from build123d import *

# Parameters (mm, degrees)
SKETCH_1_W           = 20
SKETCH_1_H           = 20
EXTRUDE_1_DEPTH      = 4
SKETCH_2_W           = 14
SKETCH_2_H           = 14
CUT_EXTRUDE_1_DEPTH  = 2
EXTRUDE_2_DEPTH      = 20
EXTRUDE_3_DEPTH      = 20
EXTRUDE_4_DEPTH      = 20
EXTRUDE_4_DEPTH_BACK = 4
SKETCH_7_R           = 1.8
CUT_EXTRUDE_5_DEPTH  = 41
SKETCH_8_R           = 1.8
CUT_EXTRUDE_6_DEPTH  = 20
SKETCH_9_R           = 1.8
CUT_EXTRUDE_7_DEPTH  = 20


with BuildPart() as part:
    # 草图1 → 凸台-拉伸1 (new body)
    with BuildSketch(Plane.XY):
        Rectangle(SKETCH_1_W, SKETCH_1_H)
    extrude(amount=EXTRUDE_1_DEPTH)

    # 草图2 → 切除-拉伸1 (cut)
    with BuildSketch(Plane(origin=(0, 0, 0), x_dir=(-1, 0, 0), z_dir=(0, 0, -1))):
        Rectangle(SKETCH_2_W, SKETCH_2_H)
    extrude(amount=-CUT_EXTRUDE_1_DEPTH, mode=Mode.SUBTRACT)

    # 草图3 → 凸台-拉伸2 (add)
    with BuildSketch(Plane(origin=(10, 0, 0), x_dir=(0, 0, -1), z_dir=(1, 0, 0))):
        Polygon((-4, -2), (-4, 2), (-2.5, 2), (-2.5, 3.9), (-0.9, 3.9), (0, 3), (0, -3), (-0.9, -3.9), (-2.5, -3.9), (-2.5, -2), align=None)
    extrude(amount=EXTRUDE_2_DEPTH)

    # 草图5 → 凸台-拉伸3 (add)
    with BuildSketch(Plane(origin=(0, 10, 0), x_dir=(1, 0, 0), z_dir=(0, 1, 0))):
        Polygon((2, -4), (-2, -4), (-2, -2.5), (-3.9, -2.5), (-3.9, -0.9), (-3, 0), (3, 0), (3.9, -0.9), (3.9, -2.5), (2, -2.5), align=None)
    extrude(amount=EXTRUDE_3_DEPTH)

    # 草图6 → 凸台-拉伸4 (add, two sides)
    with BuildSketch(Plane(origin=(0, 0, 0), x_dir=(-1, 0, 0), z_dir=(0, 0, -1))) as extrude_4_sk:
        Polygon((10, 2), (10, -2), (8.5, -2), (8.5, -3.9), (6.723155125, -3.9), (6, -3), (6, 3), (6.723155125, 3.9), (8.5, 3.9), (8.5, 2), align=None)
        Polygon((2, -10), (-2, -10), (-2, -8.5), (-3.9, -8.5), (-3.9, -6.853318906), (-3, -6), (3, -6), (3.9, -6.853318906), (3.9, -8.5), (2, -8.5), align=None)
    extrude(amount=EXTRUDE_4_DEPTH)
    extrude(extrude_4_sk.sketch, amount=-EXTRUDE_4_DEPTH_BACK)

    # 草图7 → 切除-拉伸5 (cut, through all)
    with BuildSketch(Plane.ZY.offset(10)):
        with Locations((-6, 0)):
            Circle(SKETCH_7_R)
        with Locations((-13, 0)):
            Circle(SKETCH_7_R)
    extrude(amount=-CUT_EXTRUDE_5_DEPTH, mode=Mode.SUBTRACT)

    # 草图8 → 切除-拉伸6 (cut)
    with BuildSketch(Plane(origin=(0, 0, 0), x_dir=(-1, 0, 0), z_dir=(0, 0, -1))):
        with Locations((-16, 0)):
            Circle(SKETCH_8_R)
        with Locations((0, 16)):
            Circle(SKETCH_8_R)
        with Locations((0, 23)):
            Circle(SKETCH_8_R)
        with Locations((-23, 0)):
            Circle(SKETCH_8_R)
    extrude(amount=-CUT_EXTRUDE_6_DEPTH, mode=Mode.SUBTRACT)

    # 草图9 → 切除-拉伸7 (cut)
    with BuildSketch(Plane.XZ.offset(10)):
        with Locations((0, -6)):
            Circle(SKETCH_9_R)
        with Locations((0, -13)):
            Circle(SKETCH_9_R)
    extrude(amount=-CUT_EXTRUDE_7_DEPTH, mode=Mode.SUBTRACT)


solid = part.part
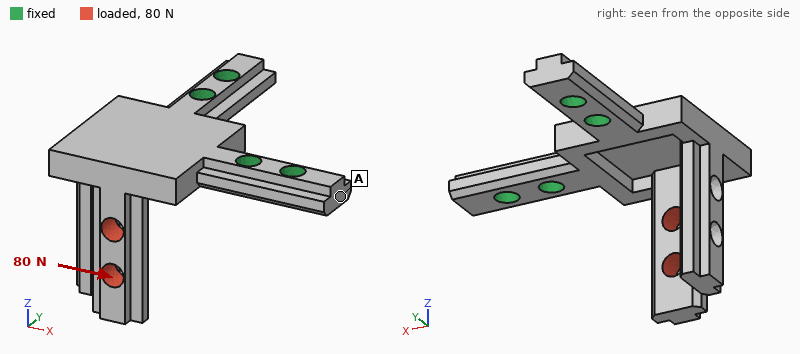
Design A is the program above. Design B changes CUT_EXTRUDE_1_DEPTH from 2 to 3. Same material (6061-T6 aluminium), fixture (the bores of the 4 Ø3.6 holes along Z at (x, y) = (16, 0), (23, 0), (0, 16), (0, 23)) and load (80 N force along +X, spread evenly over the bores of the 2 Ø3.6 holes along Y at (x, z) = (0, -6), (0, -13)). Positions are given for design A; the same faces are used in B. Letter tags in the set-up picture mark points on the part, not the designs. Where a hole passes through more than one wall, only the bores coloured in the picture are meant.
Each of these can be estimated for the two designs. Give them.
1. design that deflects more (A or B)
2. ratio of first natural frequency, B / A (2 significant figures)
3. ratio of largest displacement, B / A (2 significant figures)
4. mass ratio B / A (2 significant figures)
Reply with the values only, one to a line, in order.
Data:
B
0.94
1.2
0.94
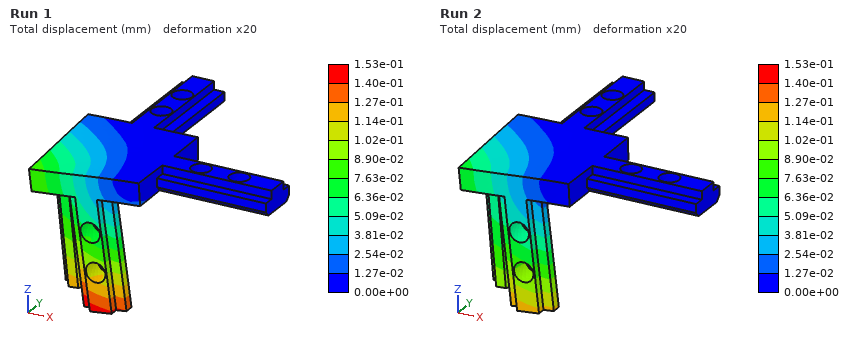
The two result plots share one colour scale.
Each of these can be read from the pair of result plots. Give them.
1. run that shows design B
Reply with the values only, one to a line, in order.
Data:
Run 1
